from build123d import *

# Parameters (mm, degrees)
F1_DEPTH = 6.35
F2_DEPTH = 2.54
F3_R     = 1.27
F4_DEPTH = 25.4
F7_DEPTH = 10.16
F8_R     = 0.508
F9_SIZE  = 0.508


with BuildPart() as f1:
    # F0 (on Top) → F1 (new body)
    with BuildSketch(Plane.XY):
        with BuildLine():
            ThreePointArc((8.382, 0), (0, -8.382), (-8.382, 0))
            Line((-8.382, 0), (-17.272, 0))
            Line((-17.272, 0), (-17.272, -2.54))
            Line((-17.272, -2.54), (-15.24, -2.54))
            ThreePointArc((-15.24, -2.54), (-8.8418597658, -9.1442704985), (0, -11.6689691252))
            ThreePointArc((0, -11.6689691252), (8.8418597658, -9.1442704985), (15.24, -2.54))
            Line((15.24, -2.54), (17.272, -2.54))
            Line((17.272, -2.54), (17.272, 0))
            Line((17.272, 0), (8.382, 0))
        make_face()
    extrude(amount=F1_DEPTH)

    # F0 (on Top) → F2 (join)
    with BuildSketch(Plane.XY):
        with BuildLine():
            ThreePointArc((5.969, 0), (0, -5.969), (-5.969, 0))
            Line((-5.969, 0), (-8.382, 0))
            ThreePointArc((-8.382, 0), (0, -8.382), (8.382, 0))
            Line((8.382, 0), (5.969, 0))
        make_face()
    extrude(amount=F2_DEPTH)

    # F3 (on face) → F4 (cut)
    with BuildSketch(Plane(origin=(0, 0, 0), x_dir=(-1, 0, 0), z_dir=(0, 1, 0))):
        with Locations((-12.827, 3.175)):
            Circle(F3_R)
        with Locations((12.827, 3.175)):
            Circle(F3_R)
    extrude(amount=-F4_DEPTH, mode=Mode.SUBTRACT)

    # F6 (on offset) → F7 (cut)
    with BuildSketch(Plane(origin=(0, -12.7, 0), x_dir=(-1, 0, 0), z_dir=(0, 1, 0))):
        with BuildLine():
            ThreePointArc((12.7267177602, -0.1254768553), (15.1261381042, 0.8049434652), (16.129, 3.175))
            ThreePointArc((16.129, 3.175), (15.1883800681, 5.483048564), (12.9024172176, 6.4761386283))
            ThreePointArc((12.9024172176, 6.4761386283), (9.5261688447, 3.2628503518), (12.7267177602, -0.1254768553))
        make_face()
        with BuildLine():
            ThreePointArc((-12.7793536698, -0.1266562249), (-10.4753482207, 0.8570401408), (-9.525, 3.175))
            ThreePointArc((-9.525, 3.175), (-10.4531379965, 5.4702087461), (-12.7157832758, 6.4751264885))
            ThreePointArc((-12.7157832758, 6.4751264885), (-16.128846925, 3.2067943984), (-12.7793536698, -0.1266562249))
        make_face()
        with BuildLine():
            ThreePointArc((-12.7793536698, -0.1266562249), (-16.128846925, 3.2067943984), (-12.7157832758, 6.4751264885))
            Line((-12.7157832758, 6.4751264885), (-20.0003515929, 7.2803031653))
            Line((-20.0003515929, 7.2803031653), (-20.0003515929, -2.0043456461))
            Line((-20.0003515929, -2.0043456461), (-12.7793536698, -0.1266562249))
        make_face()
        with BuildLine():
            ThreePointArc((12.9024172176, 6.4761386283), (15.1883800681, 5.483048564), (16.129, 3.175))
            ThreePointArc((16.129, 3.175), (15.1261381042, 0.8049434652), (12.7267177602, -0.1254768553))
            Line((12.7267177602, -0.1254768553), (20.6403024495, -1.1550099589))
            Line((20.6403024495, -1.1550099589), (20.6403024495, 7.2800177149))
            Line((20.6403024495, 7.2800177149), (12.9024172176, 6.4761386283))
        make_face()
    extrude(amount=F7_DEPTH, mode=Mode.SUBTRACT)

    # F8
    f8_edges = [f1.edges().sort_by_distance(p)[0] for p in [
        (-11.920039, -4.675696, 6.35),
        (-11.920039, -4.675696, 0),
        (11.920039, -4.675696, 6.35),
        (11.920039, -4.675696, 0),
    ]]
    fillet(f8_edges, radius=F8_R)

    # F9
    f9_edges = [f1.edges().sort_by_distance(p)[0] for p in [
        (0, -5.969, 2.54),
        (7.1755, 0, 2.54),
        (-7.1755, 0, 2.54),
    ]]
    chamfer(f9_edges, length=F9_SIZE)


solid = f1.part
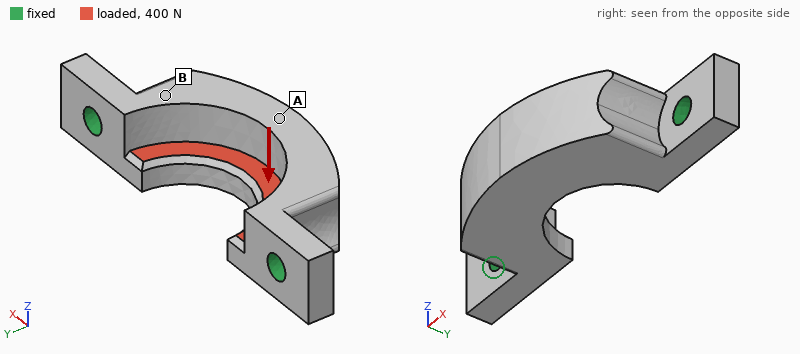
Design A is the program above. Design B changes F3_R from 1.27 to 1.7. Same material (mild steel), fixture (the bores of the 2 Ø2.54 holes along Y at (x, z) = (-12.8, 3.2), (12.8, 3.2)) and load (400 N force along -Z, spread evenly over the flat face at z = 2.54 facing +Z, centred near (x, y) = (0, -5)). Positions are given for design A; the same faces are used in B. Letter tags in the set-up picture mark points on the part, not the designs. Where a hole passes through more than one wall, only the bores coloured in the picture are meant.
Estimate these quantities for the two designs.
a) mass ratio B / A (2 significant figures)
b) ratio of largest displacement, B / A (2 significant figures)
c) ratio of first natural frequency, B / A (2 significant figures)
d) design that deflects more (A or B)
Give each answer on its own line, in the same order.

0.98
0.77
1.1
A
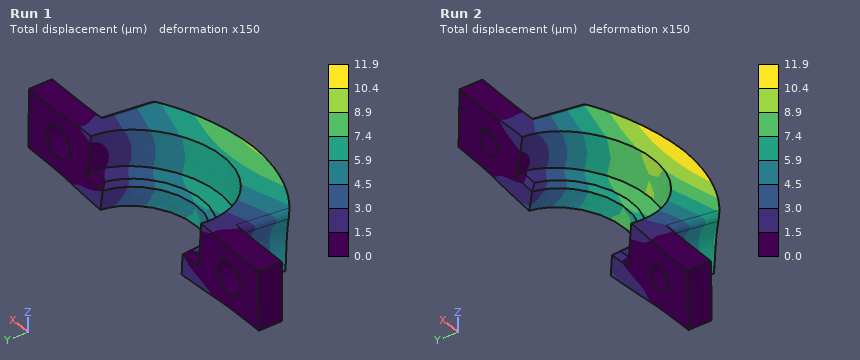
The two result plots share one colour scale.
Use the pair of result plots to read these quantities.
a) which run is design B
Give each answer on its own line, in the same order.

Run 1
